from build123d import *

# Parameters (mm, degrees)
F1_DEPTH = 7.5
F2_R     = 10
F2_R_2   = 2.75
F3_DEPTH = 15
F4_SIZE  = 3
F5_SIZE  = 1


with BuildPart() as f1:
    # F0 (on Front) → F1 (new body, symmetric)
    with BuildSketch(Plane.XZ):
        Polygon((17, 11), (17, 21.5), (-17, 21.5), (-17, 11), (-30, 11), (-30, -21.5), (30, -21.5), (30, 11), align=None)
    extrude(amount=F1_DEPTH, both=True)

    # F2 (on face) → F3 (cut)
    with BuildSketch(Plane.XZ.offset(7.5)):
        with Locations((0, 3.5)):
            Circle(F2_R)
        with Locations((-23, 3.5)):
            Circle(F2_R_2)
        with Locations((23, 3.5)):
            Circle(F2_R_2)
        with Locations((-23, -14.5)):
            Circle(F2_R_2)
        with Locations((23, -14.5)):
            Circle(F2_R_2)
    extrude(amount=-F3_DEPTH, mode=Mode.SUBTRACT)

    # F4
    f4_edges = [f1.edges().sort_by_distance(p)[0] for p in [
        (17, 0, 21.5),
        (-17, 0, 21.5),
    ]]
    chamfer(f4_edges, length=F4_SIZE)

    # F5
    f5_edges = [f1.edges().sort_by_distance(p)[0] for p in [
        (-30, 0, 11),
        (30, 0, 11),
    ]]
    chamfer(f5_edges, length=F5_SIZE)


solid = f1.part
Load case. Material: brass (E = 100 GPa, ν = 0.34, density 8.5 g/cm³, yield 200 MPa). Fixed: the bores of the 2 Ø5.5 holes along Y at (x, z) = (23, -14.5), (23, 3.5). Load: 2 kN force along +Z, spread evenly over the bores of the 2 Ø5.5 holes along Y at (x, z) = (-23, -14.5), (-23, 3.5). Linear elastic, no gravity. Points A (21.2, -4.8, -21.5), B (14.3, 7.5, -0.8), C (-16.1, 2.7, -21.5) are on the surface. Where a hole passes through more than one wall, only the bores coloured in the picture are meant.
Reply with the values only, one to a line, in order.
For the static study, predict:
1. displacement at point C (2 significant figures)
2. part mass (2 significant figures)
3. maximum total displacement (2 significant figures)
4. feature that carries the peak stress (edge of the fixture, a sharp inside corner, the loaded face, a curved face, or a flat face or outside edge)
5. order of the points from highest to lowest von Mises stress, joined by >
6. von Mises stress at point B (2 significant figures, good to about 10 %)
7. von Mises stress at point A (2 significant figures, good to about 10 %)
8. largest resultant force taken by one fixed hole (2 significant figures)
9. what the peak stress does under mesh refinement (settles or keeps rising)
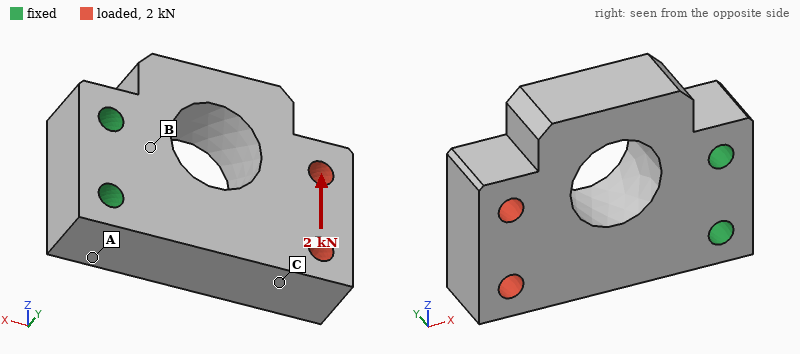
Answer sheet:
29 µm
240 g
40 µm
edge of the fixture
B > A > C
35 MPa
21 MPa
4.2 kN
keeps rising
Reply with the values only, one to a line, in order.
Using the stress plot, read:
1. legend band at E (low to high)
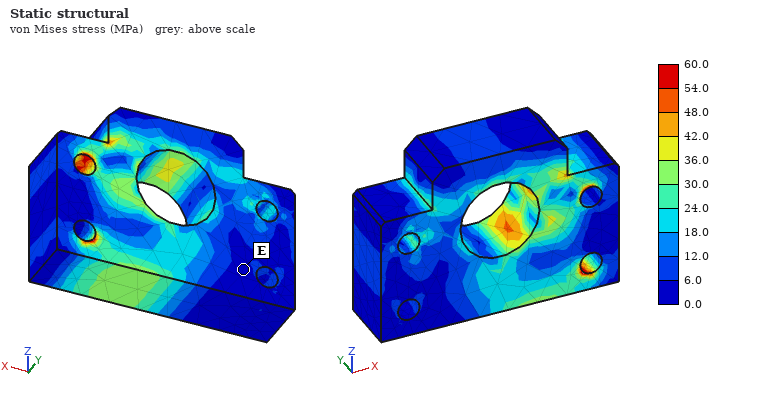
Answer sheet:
0.0 to 6.0 MPa
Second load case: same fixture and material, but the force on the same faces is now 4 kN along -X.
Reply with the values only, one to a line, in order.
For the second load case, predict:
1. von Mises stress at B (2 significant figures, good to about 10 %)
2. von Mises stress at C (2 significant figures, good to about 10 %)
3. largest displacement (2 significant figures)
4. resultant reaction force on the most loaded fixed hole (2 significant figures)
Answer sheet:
11 MPa
9.0 MPa
12 µm
2.1 kN
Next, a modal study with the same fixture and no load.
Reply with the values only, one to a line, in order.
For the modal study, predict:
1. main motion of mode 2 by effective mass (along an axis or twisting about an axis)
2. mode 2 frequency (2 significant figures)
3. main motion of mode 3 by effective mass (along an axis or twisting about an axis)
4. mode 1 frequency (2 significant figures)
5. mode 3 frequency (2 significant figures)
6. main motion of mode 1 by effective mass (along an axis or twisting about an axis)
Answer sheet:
along Z
3900 Hz
twisting about X
2600 Hz
5800 Hz
along Y
